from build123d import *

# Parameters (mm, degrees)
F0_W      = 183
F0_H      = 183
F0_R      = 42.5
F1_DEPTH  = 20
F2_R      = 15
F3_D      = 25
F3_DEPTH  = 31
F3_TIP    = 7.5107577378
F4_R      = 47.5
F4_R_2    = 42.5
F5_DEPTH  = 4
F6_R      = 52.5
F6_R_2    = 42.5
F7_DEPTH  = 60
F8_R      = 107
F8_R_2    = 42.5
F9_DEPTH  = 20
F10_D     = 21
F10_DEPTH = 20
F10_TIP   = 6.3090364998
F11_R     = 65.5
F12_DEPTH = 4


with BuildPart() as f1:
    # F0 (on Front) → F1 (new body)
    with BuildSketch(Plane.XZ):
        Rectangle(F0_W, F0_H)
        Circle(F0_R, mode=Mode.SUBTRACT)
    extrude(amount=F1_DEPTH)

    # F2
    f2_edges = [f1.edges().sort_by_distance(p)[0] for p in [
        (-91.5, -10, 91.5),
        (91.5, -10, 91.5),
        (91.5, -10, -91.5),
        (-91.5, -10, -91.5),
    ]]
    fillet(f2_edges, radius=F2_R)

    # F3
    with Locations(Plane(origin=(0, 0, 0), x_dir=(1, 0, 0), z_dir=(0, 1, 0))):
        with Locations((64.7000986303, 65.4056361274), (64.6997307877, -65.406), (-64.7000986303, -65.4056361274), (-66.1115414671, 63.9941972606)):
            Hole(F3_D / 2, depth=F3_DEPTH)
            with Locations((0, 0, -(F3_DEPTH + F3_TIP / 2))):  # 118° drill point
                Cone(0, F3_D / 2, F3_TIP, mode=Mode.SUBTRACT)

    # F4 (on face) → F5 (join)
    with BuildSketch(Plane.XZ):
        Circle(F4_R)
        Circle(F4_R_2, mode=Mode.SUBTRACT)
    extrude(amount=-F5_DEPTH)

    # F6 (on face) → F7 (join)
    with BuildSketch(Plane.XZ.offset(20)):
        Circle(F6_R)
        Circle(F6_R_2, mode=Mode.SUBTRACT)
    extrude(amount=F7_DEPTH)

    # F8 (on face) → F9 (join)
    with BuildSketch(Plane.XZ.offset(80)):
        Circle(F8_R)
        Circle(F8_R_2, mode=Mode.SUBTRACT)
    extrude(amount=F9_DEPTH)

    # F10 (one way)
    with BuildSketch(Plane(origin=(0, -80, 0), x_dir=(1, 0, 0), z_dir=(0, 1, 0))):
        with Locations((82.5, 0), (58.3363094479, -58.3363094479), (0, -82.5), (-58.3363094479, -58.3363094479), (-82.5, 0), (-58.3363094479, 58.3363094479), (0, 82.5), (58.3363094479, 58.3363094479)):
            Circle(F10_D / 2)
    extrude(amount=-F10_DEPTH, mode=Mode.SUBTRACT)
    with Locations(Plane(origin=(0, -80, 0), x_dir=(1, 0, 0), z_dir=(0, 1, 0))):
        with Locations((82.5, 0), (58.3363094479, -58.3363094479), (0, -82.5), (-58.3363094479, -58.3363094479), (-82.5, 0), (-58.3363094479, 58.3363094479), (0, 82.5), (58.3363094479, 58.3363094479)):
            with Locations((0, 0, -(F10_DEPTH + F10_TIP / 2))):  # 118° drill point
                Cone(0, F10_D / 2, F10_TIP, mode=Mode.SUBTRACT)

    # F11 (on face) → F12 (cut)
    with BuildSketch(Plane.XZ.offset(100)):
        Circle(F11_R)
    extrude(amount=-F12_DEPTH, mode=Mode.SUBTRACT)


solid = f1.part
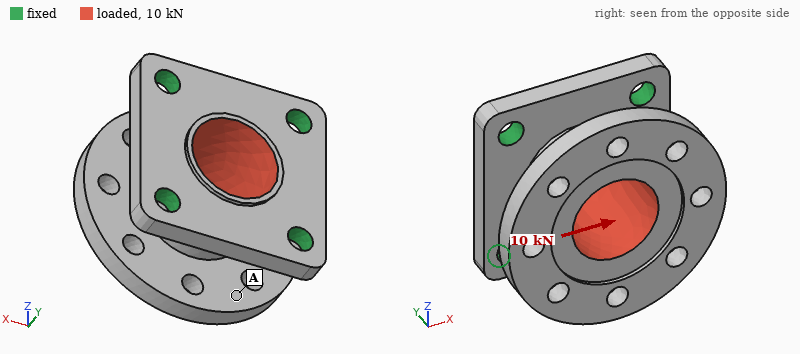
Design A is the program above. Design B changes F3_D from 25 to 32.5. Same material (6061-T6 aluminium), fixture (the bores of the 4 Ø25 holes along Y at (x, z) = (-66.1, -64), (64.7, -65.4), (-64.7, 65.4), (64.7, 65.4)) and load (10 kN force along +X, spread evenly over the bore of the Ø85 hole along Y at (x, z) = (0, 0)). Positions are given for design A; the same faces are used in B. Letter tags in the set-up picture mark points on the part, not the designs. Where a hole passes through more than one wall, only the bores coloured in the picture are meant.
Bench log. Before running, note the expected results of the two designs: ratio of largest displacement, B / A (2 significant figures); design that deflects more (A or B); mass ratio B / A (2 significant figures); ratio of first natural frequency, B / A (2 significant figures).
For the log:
0.87
A
0.98
1.0
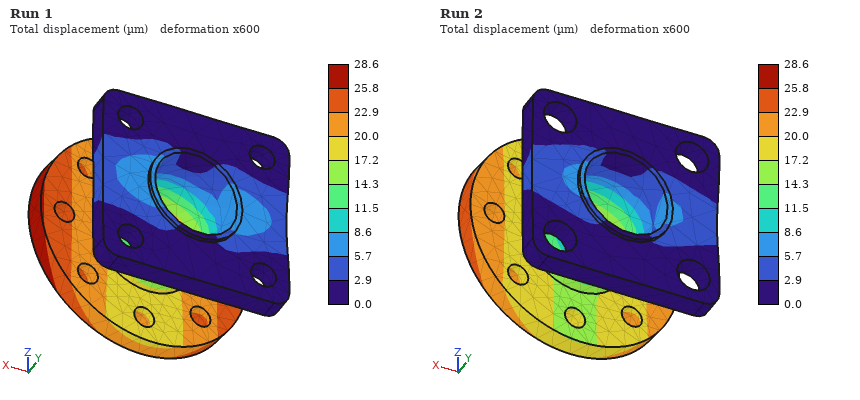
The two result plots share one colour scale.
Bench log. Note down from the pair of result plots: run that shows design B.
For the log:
Run 2
